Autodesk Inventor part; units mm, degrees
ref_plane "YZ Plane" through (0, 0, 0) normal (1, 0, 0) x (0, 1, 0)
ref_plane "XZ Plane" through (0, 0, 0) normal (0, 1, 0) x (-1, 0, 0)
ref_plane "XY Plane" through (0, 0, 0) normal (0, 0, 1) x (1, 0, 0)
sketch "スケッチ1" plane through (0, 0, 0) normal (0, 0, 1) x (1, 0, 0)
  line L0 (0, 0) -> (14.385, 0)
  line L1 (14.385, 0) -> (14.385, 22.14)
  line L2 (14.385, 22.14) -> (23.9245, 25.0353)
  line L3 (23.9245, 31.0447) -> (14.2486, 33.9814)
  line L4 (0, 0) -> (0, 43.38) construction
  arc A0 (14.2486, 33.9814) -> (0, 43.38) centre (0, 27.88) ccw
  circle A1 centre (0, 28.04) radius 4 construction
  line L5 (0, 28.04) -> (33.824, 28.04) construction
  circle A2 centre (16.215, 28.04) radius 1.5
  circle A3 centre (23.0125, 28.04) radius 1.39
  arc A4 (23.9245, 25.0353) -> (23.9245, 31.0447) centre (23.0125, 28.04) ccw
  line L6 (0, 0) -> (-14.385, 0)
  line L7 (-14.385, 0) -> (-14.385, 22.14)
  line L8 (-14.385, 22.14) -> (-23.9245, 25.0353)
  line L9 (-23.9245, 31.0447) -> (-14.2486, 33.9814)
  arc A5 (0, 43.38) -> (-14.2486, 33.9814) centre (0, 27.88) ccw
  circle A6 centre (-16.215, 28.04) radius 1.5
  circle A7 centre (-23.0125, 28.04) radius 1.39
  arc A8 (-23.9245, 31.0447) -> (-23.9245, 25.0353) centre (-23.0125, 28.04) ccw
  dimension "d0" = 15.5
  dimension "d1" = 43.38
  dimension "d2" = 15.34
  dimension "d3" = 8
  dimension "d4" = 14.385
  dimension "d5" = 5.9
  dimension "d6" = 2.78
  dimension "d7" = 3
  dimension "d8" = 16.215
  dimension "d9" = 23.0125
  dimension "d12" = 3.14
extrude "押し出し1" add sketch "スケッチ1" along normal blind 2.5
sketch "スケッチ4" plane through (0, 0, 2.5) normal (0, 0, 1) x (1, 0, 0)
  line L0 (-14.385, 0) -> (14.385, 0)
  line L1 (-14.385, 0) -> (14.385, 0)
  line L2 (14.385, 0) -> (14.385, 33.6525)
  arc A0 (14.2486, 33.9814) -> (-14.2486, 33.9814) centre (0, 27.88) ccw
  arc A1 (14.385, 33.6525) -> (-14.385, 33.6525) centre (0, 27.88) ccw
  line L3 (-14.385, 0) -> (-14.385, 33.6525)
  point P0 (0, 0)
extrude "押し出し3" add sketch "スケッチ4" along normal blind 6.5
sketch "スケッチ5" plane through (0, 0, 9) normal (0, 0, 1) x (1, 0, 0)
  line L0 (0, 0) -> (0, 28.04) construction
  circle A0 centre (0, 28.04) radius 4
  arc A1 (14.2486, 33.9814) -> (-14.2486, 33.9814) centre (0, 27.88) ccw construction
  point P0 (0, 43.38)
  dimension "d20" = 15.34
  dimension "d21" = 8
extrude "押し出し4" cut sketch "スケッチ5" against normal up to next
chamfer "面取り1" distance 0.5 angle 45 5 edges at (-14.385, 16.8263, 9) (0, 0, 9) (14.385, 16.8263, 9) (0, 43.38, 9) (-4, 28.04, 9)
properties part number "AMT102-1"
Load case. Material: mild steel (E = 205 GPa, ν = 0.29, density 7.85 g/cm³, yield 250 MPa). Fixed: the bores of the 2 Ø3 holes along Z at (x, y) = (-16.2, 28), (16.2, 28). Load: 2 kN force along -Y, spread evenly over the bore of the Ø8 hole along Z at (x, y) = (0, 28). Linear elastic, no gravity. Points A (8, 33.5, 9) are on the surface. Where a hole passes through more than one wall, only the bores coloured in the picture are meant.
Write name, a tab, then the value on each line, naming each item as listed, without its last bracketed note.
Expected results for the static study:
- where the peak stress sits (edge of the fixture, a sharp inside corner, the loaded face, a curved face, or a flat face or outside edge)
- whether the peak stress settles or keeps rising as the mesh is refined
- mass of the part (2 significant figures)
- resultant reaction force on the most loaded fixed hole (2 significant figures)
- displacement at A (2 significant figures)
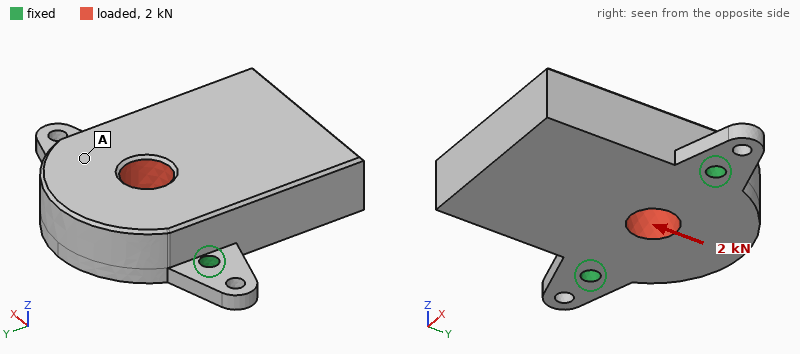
where the peak stress sits	edge of the fixture
whether the peak stress settles or keeps rising as the mesh is refined	keeps rising
mass of the part	82 g
resultant reaction force on the most loaded fixed hole	1.0 kN
displacement at A	14 µm
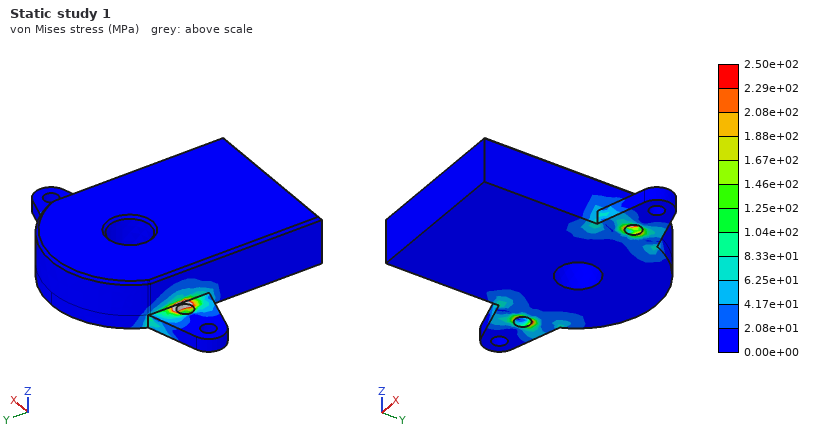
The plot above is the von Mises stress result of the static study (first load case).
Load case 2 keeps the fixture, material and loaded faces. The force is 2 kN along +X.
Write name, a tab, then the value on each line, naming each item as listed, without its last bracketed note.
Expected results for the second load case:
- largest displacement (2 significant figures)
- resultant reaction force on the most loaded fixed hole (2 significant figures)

largest displacement	1.6 µm
resultant reaction force on the most loaded fixed hole	1.0 kN
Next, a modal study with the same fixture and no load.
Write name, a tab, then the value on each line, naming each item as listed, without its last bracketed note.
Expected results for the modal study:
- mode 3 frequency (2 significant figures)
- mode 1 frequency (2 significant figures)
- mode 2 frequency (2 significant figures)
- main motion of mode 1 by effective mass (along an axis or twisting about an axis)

mode 3 frequency	14 kHz
mode 1 frequency	2500 Hz
mode 2 frequency	13 kHz
main motion of mode 1 by effective mass	along Z
